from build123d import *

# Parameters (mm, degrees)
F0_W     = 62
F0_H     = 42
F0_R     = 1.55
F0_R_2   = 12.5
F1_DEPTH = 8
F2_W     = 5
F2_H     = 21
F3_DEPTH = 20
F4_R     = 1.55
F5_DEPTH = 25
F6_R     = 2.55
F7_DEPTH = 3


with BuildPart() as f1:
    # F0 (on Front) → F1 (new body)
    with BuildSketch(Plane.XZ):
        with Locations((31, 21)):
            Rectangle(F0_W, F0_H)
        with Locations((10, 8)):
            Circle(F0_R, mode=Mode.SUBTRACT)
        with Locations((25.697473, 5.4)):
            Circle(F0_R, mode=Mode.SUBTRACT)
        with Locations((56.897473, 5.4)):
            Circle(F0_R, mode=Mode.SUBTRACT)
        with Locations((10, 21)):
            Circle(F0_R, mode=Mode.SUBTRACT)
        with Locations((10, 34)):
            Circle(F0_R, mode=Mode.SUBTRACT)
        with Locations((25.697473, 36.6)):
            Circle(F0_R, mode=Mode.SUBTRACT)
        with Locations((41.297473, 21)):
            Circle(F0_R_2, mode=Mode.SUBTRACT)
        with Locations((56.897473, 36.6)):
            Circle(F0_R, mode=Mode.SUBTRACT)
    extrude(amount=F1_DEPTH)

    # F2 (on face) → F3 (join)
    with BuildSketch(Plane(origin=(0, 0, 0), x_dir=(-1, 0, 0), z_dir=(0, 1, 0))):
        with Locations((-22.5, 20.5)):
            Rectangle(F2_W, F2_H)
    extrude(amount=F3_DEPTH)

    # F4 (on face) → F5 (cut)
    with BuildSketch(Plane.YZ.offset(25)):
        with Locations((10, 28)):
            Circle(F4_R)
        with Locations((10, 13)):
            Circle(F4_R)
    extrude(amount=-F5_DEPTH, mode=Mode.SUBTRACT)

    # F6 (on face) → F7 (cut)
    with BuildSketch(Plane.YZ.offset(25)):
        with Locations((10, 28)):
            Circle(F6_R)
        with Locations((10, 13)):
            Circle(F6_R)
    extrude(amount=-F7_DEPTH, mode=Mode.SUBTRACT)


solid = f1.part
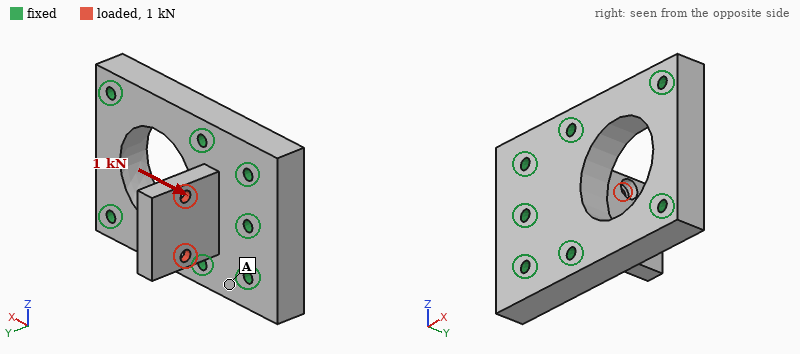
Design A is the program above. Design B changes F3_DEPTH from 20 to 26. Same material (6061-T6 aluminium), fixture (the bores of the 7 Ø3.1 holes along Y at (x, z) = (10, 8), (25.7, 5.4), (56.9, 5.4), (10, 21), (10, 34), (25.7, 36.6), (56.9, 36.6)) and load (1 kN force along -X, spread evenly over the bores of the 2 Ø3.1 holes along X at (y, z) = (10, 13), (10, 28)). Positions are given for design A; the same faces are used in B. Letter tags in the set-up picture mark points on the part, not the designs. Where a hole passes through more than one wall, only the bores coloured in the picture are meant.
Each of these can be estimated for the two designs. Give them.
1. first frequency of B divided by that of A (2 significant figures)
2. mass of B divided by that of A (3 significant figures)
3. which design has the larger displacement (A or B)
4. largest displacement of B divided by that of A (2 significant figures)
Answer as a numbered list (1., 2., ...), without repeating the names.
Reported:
1. 0.61
2. 1.03
3. B
4. 1.3
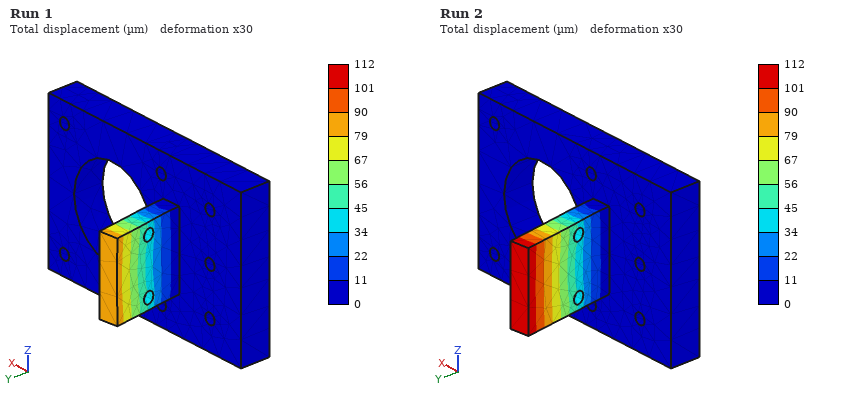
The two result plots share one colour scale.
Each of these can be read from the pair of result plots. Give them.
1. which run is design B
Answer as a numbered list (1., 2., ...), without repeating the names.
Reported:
1. Run 2
